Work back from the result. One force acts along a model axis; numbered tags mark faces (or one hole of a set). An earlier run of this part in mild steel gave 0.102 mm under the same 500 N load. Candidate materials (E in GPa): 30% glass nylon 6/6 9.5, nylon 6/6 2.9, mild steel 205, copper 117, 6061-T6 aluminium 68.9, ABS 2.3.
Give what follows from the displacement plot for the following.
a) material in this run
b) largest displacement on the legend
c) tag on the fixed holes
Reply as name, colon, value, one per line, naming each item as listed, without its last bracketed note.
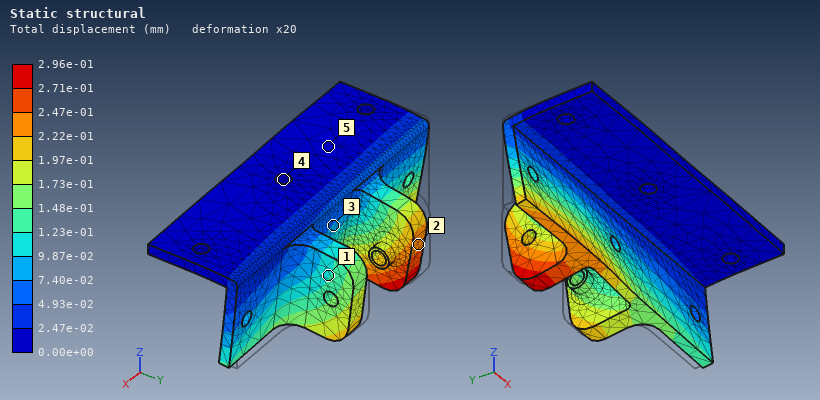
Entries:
material in this run: 6061-T6 aluminium
largest displacement on the legend: 2.96e-01 mm
tag on the fixed holes: 4
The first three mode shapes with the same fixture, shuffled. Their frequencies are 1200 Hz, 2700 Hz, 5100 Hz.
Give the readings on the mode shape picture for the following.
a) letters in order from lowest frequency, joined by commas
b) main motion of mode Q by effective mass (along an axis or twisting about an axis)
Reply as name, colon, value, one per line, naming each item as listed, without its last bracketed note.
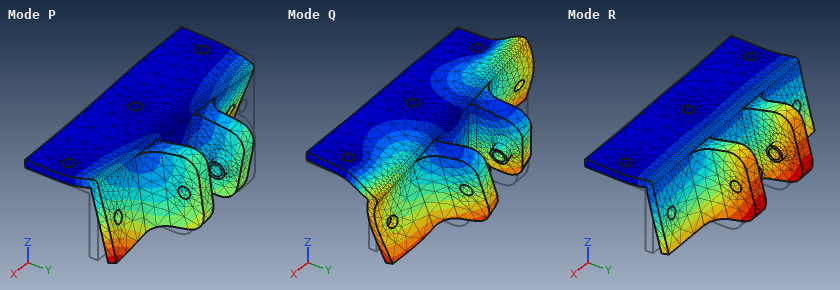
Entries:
letters in order from lowest frequency, joined by commas: R, P, Q
main motion of mode Q by effective mass: along X
